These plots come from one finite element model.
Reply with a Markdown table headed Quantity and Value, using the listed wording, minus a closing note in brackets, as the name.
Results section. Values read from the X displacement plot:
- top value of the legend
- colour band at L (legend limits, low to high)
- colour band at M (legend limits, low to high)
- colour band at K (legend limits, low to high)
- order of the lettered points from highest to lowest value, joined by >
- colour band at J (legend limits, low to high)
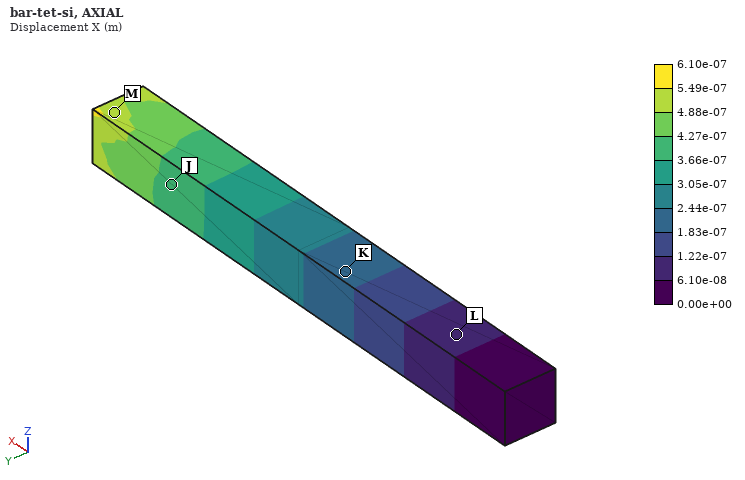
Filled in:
| Quantity | Value |
|---|---|
| top value of the legend | 6.10e-07 m |
| colour band at L | 6.10e-08 to 1.22e-07 m |
| colour band at M | 4.88e-07 to 5.49e-07 m |
| colour band at K | 1.83e-07 to 2.44e-07 m |
| order of the lettered points from highest to lowest value, joined by > | M > J > K > L |
| colour band at J | 3.66e-07 to 4.27e-07 m |
